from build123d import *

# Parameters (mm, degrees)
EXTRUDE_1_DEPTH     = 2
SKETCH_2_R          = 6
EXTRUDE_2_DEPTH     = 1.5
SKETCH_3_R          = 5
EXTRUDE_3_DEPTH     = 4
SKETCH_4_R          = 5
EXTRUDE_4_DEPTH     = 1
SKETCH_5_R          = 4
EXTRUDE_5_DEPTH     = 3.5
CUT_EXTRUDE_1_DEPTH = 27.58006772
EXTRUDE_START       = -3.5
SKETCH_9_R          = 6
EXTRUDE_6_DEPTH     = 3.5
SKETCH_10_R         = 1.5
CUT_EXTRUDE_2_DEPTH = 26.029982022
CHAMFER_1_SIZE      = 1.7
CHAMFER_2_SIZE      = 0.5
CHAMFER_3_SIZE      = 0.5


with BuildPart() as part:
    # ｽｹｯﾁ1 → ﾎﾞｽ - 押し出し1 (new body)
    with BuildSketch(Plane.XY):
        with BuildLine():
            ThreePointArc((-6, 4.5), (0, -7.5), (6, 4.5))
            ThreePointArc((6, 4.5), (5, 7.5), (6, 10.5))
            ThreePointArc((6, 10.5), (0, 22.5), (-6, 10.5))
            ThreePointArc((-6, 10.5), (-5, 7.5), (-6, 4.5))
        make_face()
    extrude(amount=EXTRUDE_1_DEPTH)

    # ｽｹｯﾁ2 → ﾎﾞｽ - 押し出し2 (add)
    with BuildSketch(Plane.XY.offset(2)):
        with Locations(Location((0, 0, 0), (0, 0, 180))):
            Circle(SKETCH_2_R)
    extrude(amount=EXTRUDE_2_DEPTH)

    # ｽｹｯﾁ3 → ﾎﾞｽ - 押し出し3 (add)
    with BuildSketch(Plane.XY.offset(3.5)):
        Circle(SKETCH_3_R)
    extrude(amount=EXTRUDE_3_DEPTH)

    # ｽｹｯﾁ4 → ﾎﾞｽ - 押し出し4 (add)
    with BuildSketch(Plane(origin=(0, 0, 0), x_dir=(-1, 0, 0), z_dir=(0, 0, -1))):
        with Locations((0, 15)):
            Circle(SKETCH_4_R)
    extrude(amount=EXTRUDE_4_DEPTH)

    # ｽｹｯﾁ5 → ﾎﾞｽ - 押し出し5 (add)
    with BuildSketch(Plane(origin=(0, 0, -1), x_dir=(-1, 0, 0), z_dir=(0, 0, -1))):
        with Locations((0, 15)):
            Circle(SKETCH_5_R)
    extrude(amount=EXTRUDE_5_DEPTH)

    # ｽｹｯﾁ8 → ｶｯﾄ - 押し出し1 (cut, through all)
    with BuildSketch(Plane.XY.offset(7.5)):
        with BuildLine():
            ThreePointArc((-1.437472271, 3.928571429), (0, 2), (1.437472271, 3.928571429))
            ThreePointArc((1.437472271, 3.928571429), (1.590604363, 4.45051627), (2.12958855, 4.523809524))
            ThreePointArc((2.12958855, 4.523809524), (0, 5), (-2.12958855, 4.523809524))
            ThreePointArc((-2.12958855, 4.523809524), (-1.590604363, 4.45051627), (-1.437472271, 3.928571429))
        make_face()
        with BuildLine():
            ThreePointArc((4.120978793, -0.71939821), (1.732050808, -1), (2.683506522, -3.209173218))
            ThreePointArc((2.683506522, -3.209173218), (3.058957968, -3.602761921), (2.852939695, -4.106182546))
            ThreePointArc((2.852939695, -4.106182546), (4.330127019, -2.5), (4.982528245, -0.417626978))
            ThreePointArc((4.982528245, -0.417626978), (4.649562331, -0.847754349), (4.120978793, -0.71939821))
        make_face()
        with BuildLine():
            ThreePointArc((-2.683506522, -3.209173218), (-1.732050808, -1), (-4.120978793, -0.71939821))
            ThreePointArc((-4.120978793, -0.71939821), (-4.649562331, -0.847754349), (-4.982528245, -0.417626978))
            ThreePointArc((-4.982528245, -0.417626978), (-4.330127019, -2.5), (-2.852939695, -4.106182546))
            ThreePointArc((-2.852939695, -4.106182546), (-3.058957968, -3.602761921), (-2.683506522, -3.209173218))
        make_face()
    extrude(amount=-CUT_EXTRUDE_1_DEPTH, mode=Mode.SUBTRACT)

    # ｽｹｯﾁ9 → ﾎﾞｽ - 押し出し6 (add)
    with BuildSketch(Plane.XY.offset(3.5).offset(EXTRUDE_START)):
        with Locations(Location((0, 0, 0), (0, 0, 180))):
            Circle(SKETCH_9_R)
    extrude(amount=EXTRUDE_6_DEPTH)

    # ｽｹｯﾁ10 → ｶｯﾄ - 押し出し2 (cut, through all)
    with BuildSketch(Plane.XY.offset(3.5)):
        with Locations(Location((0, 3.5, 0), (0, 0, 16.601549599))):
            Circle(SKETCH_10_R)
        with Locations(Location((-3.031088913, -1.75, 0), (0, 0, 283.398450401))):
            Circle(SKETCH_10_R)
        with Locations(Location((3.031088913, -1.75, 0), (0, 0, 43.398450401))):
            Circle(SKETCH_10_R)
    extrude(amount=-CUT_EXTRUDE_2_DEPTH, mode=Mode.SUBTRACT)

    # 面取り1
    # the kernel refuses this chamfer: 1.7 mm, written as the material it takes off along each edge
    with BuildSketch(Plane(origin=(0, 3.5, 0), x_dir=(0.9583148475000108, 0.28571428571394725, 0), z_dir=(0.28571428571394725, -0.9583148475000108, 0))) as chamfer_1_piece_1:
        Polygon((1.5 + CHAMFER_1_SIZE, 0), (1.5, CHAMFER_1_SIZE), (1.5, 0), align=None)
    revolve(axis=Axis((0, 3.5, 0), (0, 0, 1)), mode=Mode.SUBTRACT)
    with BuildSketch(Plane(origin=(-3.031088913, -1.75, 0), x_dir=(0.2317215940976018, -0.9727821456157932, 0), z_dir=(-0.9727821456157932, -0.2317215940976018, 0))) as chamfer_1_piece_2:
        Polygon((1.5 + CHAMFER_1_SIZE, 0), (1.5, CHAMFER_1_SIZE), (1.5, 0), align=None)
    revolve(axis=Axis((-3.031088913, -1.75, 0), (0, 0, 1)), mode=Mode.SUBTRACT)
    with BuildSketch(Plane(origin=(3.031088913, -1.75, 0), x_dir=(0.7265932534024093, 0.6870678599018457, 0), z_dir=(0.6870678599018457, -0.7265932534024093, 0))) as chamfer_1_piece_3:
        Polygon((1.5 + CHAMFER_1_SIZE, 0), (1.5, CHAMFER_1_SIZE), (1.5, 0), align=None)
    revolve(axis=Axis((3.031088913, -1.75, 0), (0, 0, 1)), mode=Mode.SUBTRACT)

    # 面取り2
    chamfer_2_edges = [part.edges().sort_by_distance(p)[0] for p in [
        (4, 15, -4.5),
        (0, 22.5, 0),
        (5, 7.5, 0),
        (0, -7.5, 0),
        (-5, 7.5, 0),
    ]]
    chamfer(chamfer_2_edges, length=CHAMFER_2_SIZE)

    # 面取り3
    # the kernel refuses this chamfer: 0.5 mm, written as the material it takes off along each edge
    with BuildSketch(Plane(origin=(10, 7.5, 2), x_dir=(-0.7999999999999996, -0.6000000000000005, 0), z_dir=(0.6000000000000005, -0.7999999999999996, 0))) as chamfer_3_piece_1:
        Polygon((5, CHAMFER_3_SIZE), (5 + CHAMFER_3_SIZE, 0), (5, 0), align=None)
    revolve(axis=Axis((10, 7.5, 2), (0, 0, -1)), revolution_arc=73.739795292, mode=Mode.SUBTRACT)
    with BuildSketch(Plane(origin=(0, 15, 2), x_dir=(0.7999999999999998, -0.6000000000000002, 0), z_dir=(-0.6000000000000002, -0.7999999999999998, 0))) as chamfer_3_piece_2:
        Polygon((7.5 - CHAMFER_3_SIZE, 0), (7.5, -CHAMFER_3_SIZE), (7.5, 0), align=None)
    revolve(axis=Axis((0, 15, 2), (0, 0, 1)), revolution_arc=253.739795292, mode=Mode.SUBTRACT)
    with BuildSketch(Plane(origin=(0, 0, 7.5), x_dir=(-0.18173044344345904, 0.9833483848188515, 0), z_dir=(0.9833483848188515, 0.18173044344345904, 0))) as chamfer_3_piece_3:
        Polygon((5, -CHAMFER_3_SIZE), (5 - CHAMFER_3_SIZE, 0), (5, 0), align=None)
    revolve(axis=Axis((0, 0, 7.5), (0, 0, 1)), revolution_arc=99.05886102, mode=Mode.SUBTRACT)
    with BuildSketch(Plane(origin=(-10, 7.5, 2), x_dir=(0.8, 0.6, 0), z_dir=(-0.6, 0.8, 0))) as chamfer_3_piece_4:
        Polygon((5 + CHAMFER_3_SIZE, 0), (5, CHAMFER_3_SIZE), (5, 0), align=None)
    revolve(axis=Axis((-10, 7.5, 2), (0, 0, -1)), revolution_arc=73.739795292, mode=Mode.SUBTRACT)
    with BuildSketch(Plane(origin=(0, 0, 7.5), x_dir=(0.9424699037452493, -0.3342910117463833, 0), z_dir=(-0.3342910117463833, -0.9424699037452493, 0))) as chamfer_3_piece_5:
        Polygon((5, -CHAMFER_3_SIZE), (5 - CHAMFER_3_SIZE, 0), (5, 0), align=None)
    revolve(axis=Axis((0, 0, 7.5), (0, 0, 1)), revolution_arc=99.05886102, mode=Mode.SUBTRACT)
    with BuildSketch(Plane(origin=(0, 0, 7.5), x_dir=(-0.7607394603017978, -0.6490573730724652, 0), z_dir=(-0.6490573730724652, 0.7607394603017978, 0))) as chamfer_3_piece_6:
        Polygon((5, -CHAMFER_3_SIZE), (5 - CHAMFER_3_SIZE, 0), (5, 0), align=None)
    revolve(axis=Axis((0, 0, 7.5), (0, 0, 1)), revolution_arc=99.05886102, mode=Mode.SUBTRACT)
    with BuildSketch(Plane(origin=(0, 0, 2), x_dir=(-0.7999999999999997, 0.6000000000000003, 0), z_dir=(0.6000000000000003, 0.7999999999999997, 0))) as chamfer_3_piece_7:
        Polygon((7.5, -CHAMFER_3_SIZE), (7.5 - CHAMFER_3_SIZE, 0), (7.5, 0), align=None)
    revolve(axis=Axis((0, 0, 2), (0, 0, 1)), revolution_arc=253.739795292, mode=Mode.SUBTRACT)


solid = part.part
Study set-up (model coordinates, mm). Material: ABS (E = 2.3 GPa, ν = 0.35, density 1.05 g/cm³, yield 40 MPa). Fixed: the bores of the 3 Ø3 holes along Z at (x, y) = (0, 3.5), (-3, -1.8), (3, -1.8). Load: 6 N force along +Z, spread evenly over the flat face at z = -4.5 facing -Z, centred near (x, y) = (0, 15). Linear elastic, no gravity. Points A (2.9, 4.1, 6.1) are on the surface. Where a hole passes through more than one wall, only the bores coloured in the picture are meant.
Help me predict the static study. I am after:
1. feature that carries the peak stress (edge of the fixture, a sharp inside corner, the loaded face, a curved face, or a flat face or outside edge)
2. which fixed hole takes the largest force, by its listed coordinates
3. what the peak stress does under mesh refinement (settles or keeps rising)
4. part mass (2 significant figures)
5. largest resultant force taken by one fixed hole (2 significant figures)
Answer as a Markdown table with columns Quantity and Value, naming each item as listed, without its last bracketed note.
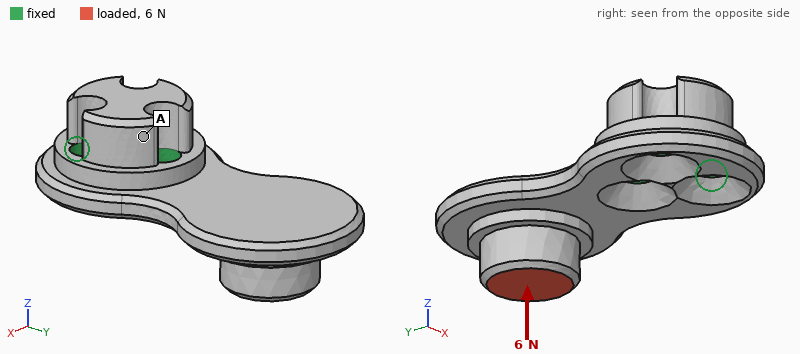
| Quantity | Value |
|---|---|
| feature that carries the peak stress | a sharp inside corner |
| which fixed hole takes the largest force, by its listed coordinates | (0, 3.5) |
| what the peak stress does under mesh refinement | keeps rising |
| part mass | 1.3 g |
| largest resultant force taken by one fixed hole | 18 N |
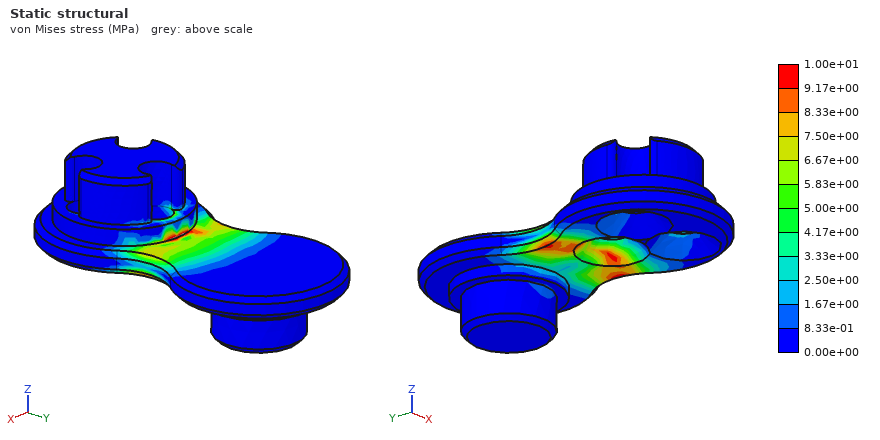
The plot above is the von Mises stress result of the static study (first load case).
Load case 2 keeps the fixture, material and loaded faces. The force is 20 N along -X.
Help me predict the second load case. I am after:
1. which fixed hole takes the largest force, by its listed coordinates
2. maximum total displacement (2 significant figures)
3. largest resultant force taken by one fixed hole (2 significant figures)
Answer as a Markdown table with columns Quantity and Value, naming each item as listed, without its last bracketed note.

| Quantity | Value |
|---|---|
| which fixed hole takes the largest force, by its listed coordinates | (0, 3.5) |
| maximum total displacement | 0.20 mm |
| largest resultant force taken by one fixed hole | 31 N |
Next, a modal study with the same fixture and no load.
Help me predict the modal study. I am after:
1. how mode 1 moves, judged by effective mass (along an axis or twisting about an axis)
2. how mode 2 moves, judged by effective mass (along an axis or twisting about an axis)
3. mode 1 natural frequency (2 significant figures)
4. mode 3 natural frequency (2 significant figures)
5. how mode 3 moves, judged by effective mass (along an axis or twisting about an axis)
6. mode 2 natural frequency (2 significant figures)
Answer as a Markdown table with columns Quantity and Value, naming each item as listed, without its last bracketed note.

| Quantity | Value |
|---|---|
| how mode 1 moves, judged by effective mass | along Z |
| how mode 2 moves, judged by effective mass | along X |
| mode 1 natural frequency | 1000 Hz |
| mode 3 natural frequency | 4200 Hz |
| how mode 3 moves, judged by effective mass | along X |
| mode 2 natural frequency | 3300 Hz |
